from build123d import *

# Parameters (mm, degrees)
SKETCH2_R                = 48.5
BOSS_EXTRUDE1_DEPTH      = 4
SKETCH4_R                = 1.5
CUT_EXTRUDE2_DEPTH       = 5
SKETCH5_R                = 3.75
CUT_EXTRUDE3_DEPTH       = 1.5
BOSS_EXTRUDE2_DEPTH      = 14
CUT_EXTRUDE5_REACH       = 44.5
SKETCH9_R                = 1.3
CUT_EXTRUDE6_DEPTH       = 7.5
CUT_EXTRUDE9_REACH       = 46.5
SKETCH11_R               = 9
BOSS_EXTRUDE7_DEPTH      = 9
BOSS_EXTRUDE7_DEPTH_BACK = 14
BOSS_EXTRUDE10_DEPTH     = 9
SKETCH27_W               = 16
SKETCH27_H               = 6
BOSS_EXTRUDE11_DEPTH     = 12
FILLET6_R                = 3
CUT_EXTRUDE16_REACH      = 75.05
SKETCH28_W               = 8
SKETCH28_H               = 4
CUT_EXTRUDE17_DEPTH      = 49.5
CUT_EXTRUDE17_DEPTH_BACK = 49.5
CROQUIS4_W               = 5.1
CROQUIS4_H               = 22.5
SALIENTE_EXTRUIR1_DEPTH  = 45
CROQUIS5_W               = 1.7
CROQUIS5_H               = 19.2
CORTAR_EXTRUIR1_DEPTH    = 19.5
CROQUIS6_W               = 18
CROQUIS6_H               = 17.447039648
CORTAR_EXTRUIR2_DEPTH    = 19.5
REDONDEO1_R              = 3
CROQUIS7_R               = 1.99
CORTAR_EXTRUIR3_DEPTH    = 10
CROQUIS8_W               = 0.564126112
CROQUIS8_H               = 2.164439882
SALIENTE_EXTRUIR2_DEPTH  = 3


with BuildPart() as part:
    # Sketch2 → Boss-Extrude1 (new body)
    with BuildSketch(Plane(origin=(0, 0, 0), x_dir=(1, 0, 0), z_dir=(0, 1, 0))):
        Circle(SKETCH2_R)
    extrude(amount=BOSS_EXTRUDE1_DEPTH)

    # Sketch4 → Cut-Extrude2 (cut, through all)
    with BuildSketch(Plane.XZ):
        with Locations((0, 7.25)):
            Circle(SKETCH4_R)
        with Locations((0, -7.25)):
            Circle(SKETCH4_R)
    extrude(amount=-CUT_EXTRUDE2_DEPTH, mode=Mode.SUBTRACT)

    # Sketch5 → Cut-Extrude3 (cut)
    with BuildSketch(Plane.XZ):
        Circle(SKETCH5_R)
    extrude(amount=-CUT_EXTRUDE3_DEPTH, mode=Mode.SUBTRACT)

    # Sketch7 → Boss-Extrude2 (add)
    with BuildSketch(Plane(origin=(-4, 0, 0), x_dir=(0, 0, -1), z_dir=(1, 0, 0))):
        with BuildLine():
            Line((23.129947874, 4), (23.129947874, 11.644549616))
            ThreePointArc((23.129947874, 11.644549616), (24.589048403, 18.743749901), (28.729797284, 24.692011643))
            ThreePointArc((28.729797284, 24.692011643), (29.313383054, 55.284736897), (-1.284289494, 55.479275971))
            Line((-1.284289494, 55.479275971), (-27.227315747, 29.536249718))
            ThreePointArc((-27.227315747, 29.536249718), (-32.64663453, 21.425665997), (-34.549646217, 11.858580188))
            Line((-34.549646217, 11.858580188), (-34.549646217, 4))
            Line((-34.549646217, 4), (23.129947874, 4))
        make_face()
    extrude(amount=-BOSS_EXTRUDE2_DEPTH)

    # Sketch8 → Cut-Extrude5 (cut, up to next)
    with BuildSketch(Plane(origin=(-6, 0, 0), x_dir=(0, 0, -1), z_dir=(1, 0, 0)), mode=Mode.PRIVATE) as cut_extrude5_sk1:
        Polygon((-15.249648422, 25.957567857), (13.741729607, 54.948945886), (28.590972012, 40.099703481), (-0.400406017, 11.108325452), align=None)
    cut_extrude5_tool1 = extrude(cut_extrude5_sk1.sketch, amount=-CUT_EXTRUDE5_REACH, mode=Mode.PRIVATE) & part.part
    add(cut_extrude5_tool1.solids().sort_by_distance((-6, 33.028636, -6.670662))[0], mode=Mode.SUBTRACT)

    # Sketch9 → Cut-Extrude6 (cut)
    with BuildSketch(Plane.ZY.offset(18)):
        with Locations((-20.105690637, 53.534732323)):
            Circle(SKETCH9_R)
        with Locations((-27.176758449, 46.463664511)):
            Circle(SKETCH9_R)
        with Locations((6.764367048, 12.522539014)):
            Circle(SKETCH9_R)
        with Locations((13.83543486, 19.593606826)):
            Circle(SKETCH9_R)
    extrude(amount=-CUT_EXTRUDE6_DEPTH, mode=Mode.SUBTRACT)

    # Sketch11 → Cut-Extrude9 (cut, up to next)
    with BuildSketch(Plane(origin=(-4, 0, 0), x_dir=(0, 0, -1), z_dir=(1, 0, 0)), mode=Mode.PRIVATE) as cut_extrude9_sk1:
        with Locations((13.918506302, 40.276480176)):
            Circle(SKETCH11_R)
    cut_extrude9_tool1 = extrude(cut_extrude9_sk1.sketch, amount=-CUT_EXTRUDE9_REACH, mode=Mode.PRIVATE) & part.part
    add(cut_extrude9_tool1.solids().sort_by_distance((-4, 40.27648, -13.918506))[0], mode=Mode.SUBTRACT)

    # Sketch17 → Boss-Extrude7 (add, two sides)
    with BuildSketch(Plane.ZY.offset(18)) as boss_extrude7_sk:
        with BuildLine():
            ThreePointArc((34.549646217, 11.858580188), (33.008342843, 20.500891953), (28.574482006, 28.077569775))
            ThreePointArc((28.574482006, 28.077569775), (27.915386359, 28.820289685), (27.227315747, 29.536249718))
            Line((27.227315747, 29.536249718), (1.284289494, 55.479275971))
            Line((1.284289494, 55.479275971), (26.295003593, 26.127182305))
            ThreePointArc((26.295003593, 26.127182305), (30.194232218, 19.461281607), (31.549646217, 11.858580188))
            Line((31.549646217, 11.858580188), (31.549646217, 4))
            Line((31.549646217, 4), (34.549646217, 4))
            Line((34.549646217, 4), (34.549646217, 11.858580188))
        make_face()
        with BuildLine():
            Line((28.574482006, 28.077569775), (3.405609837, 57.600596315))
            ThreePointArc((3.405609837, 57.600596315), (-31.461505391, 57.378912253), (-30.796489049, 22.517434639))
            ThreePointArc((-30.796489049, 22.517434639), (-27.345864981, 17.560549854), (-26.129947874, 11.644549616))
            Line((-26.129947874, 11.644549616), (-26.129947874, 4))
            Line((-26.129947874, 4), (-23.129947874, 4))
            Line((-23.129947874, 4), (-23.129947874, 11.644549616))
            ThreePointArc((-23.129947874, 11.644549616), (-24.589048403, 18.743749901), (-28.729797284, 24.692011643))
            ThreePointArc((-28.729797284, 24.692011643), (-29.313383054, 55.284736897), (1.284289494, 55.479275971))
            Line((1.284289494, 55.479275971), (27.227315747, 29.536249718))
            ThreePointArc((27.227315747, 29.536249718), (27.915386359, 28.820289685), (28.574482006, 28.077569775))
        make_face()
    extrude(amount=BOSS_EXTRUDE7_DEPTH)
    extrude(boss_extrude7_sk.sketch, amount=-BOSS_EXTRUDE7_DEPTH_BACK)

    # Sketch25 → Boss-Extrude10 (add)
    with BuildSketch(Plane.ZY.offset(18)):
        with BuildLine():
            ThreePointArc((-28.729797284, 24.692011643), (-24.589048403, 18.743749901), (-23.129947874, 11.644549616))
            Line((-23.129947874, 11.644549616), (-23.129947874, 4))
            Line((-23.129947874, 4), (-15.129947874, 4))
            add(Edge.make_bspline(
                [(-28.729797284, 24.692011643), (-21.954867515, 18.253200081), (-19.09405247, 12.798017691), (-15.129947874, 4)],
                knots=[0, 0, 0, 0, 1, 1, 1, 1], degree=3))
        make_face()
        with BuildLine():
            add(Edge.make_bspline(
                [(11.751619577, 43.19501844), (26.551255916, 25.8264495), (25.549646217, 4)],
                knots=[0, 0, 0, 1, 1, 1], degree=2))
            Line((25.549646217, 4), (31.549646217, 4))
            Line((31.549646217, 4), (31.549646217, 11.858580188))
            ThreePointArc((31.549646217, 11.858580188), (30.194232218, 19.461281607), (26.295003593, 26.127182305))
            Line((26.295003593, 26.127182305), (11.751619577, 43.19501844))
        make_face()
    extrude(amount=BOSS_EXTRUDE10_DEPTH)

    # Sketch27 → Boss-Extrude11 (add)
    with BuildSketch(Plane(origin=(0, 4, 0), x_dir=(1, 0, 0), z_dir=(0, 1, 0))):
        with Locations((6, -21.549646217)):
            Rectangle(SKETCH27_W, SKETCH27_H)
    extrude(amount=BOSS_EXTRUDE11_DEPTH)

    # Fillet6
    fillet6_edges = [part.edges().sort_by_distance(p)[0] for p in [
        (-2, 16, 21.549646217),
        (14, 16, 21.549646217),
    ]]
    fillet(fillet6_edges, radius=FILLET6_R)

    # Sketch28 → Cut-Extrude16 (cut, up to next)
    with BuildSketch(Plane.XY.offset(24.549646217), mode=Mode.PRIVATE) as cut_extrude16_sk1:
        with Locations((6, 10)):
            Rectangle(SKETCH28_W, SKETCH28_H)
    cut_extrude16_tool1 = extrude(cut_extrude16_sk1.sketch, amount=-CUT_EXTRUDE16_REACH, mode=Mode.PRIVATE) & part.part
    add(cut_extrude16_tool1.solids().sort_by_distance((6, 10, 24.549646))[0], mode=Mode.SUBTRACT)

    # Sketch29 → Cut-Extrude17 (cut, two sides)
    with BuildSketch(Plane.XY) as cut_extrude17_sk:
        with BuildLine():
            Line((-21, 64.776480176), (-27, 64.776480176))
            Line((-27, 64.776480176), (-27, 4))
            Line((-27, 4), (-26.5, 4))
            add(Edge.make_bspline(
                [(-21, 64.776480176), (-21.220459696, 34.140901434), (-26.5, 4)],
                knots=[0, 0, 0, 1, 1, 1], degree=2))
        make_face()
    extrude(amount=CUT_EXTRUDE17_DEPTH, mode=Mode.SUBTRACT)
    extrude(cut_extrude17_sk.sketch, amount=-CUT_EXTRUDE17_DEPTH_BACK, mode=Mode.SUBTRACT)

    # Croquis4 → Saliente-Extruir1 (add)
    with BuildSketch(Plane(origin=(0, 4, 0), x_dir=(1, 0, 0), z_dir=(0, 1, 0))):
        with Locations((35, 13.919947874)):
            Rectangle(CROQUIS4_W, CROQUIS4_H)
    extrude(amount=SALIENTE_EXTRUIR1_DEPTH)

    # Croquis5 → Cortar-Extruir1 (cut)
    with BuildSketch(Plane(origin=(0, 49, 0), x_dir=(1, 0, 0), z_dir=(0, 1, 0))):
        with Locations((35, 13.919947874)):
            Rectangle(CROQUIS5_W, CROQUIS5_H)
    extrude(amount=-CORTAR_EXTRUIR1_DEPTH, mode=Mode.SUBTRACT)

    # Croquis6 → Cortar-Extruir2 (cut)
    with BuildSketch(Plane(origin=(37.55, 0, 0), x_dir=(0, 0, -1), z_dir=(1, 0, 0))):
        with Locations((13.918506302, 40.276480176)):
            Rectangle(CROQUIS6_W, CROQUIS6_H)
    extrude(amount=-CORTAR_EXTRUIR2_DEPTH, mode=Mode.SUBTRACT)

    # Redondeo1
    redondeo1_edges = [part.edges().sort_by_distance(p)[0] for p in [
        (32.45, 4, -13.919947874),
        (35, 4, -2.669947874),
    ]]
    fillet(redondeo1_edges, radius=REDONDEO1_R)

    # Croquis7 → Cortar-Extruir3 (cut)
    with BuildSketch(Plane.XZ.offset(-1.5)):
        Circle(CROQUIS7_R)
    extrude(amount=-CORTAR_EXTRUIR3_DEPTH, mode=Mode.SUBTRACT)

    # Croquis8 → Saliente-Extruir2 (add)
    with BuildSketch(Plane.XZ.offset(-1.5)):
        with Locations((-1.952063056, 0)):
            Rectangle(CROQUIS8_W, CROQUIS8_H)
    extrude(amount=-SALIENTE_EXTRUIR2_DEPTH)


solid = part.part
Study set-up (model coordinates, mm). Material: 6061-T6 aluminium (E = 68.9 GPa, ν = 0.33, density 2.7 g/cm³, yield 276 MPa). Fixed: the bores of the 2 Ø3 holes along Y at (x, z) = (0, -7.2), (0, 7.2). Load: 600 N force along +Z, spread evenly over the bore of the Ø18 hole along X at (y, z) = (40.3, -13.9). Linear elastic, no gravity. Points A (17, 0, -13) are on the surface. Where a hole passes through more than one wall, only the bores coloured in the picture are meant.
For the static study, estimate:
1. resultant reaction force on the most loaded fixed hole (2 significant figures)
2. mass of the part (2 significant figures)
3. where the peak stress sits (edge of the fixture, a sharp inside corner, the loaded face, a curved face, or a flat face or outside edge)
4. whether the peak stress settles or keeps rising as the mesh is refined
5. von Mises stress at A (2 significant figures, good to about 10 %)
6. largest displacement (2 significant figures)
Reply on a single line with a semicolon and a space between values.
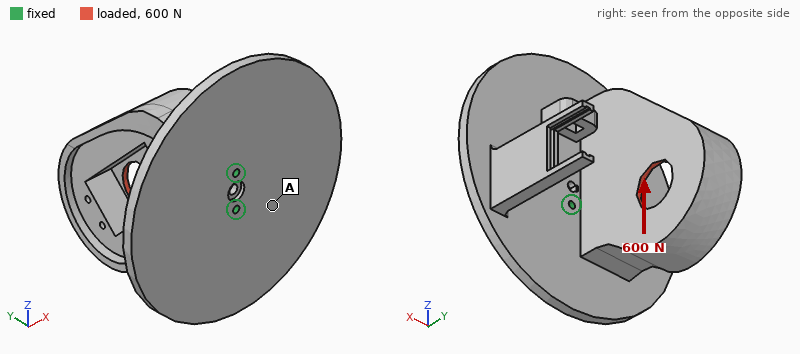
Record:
1.3 kN; 190 g; edge of the fixture; keeps rising; 7.7 MPa; 0.10 mm
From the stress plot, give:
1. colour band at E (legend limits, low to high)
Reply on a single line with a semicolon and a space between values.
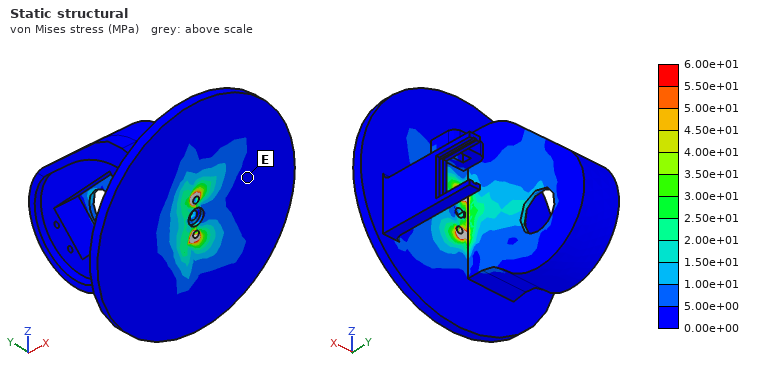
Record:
0.00e+00 to 5.00e+00 MPa
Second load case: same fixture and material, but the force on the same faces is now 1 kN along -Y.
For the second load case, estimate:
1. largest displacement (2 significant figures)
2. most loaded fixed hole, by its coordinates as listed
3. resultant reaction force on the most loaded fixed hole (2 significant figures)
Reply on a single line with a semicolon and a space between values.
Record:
92 µm; (0, -7.2); 1.2 kN
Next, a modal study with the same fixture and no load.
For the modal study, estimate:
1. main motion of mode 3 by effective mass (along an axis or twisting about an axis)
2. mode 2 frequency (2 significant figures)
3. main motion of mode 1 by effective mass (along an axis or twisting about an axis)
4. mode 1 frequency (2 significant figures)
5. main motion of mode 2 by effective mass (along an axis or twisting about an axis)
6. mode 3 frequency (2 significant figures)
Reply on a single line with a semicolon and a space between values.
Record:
along Z; 1200 Hz; along X; 630 Hz; along Y; 1400 Hz
